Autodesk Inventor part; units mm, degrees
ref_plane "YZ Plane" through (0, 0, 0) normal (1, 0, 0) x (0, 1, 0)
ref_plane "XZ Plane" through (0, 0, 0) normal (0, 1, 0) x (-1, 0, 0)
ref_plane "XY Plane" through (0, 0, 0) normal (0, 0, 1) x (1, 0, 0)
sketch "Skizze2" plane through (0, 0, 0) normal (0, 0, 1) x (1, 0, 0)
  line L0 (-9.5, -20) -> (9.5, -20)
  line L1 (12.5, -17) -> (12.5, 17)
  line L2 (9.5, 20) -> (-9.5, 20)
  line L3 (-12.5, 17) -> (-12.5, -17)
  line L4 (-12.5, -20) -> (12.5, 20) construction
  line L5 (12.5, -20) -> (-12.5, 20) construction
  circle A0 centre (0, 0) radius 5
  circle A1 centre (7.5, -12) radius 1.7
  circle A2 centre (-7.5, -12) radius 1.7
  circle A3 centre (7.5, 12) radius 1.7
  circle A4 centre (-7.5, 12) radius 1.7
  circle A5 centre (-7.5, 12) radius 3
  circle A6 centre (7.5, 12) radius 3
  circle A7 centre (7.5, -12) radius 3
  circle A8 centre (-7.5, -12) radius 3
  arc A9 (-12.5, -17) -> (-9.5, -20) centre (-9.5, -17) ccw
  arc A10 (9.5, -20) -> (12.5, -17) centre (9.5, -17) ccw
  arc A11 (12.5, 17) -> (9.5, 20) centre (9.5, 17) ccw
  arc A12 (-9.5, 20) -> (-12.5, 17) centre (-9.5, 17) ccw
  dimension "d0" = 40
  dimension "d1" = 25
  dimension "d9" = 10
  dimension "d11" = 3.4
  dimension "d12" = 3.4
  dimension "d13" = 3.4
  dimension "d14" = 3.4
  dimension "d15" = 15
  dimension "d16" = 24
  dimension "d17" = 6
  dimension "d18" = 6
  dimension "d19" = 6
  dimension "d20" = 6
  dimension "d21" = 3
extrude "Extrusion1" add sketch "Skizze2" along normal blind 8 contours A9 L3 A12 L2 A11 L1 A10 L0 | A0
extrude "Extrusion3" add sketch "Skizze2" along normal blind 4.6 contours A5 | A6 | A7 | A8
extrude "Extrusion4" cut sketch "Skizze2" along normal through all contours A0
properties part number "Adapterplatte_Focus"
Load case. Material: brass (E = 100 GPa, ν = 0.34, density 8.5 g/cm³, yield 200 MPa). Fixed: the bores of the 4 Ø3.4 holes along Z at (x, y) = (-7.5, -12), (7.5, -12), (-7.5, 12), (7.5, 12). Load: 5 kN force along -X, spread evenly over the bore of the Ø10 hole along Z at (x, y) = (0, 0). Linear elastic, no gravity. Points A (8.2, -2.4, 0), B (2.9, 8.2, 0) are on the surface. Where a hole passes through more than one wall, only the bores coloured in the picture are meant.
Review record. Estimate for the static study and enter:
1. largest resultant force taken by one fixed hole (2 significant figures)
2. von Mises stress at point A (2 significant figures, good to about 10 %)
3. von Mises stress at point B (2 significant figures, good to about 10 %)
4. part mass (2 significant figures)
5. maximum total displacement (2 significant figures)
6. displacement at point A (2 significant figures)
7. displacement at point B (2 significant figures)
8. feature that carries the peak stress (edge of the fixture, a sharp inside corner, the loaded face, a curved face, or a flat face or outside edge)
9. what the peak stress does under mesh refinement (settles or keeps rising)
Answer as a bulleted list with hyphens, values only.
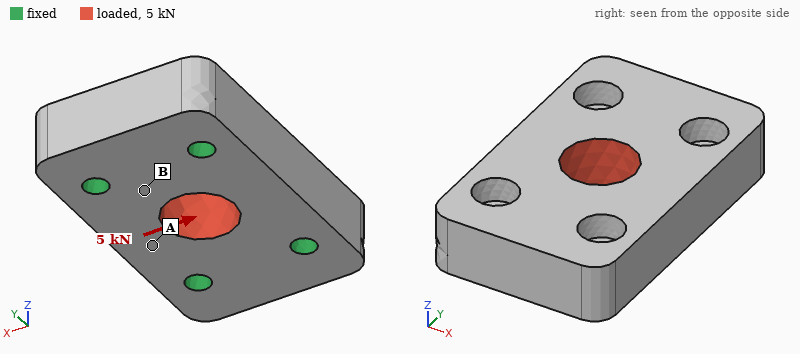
- 1.4 kN
- 18 MPa
- 33 MPa
- 57 g
- 5.8 µm
- 4.2 µm
- 1.9 µm
- edge of the fixture
- keeps rising
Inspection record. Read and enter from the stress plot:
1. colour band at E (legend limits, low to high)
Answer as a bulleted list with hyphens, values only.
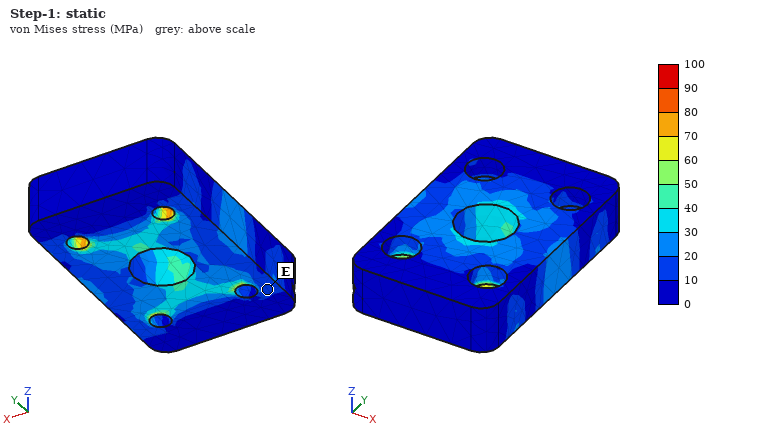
- 10 to 20 MPa
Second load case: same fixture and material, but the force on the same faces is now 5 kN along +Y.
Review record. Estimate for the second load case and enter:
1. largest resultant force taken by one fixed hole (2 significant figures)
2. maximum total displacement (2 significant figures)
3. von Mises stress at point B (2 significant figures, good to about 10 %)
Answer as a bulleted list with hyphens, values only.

- 1.3 kN
- 3.1 µm
- 18 MPa
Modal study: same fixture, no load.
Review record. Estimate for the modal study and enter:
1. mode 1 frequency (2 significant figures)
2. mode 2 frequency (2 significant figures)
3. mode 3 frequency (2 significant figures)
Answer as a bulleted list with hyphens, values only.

- 24 kHz
- 29 kHz
- 29 kHz
